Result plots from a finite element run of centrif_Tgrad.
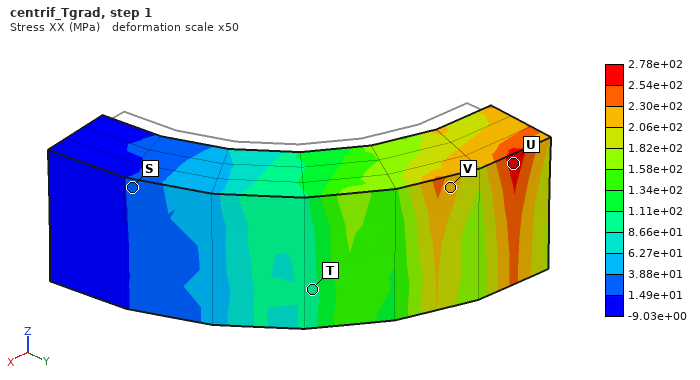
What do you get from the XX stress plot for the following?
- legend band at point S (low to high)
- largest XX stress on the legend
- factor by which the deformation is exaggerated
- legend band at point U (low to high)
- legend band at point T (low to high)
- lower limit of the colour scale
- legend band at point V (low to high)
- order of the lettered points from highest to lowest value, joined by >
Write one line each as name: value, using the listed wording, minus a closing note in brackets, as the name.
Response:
legend band at point S: 1.49e+01 to 3.88e+01 MPa
largest XX stress on the legend: 2.78e+02 MPa
factor by which the deformation is exaggerated: 50
legend band at point U: 2.54e+02 to 2.78e+02 MPa
legend band at point T: 8.66e+01 to 1.11e+02 MPa
lower limit of the colour scale: -9.03e+00 MPa
legend band at point V: 2.06e+02 to 2.30e+02 MPa
order of the lettered points from highest to lowest value, joined by >: U > V > T > S
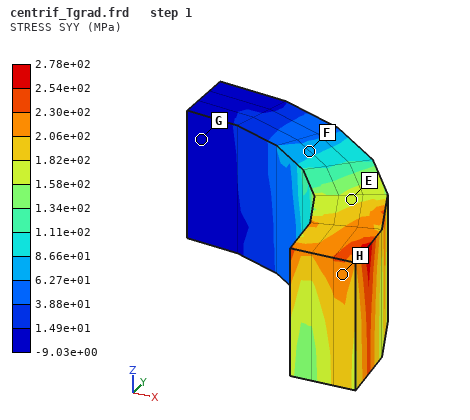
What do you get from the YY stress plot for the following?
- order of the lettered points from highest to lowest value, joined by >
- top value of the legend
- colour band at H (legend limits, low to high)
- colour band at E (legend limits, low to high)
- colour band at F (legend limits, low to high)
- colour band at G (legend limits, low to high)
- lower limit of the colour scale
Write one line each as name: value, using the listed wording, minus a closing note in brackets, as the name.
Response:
order of the lettered points from highest to lowest value, joined by >: H > E > F > G
top value of the legend: 2.78e+02 MPa
colour band at H: 2.06e+02 to 2.30e+02 MPa
colour band at E: 1.58e+02 to 1.82e+02 MPa
colour band at F: 6.27e+01 to 8.66e+01 MPa
colour band at G: -9.03e+00 to 1.49e+01 MPa
lower limit of the colour scale: -9.03e+00 MPa
